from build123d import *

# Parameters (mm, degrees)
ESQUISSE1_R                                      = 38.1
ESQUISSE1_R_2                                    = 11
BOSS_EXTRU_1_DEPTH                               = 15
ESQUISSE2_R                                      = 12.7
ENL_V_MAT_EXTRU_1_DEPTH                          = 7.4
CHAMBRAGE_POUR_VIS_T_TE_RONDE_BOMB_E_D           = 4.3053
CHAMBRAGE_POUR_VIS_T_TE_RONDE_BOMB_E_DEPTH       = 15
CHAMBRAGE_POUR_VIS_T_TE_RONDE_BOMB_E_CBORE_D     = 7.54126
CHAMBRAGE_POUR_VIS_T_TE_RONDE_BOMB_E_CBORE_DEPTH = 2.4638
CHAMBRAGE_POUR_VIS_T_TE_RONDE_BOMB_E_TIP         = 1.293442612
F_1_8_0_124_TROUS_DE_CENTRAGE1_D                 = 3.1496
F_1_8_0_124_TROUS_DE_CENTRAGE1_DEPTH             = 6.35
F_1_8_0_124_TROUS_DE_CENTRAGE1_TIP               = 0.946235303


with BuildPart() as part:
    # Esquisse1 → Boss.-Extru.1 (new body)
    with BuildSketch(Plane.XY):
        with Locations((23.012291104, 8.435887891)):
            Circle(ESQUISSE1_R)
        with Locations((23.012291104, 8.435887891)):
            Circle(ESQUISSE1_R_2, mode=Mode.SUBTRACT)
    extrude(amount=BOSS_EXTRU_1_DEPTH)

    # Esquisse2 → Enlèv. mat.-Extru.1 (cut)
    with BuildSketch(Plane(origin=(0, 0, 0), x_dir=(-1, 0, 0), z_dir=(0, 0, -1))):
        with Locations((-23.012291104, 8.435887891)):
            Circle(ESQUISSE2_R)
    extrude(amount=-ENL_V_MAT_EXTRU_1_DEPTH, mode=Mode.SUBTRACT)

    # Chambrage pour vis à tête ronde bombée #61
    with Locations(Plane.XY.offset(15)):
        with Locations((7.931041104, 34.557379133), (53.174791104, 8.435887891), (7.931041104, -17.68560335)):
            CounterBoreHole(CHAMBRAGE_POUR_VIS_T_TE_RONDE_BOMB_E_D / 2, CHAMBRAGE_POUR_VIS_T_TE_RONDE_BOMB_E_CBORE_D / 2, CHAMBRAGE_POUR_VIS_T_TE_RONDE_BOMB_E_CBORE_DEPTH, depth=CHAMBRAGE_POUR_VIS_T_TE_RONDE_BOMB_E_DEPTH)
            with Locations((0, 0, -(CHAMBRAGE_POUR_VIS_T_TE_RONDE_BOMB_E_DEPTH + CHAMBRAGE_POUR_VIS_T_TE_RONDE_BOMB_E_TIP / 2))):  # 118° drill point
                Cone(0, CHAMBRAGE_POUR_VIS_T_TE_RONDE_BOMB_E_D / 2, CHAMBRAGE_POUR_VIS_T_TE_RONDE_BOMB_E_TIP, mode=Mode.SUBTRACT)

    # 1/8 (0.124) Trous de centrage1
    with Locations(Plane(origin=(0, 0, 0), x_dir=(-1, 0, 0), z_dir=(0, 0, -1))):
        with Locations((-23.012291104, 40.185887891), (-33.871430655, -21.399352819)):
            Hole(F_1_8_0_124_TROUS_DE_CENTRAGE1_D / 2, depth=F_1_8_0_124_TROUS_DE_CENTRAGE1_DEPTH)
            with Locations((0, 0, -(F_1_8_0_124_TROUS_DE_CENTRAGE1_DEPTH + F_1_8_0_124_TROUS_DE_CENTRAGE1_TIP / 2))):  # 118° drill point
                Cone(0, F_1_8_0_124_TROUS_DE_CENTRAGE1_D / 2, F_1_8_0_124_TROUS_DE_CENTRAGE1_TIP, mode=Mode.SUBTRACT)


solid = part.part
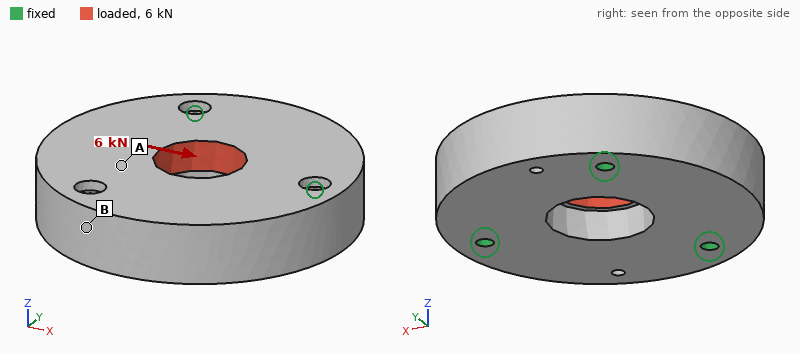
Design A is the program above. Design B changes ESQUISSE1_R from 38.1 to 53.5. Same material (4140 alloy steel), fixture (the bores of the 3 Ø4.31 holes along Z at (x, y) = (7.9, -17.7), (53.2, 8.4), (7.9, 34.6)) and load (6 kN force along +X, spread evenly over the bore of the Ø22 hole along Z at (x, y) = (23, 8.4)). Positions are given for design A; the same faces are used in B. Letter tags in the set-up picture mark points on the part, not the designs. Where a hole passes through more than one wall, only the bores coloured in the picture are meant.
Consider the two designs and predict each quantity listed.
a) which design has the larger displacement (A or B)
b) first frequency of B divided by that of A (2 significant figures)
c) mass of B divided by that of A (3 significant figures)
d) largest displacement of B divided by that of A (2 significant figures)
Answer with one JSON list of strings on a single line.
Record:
["A", "0.53", "2.09", "0.83"]
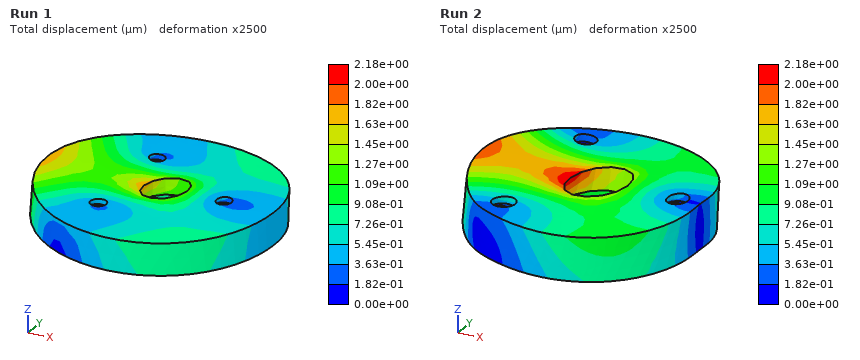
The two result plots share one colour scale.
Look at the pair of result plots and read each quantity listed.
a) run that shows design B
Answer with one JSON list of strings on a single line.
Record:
["Run 1"]
